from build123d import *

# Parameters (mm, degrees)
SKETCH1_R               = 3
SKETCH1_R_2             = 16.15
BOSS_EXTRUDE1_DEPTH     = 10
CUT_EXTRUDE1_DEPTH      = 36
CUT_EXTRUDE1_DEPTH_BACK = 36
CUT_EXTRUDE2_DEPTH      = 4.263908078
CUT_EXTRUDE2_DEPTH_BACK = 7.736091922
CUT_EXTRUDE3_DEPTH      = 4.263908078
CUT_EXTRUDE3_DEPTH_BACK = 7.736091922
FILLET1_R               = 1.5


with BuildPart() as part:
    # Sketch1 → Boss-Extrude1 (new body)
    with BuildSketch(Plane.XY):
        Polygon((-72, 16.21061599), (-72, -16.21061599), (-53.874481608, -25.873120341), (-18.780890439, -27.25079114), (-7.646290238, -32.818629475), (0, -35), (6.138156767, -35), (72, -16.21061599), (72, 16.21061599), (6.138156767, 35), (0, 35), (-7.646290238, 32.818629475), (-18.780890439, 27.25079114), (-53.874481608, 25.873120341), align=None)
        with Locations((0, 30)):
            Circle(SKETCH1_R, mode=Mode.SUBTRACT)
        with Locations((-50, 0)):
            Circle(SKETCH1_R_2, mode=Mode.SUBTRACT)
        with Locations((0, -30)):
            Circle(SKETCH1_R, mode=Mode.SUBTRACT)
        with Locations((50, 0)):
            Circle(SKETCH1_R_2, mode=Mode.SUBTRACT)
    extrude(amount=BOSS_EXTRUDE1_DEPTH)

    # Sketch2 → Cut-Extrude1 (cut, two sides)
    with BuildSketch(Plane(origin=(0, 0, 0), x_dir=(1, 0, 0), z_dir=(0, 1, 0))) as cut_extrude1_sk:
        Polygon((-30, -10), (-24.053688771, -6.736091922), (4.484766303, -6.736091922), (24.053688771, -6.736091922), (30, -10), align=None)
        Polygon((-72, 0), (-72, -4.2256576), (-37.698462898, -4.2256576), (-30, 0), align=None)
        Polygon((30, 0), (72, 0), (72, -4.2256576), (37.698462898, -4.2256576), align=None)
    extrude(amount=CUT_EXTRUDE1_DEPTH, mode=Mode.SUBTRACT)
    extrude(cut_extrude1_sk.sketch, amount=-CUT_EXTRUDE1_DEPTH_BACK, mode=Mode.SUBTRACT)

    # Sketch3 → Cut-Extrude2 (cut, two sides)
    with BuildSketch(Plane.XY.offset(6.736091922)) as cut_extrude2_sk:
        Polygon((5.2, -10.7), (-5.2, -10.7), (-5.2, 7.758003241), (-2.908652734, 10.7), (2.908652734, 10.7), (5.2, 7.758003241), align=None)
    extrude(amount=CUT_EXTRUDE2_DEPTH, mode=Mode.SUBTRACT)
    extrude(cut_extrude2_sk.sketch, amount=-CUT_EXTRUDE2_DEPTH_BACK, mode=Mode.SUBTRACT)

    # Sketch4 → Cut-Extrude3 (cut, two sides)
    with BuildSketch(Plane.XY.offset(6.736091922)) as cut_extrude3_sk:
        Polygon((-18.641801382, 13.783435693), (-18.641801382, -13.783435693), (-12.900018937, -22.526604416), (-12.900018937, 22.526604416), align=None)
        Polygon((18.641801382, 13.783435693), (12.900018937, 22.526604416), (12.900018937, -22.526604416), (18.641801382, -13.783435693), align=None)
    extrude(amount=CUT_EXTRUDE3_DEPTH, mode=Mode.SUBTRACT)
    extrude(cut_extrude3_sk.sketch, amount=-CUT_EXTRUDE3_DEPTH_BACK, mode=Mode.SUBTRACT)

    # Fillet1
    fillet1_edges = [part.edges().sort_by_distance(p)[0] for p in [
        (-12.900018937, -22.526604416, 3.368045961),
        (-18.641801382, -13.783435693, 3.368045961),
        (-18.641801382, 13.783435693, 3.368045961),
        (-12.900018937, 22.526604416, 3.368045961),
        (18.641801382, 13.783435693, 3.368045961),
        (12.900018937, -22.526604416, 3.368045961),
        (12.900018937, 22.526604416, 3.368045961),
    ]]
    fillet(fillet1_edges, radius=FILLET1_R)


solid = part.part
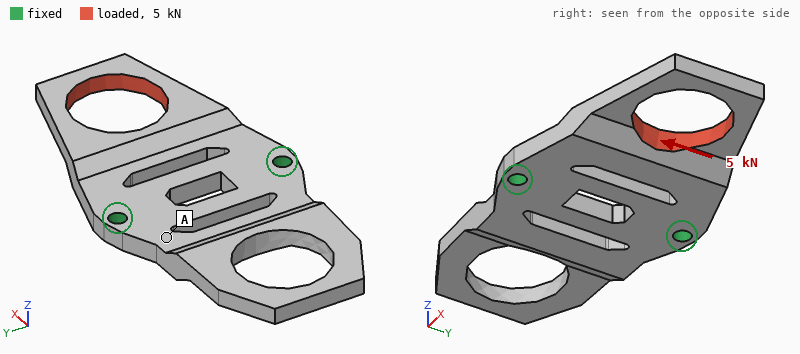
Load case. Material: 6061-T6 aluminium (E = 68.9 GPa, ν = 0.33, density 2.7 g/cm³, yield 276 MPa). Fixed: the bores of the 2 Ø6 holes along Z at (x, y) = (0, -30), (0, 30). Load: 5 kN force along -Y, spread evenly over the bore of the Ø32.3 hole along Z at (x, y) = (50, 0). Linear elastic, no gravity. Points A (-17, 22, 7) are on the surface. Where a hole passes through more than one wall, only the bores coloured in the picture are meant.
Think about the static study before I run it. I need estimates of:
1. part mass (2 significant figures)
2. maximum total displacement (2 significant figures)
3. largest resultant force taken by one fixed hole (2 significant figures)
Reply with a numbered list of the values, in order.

1. 98 g
2. 0.22 mm
3. 4.5 kN
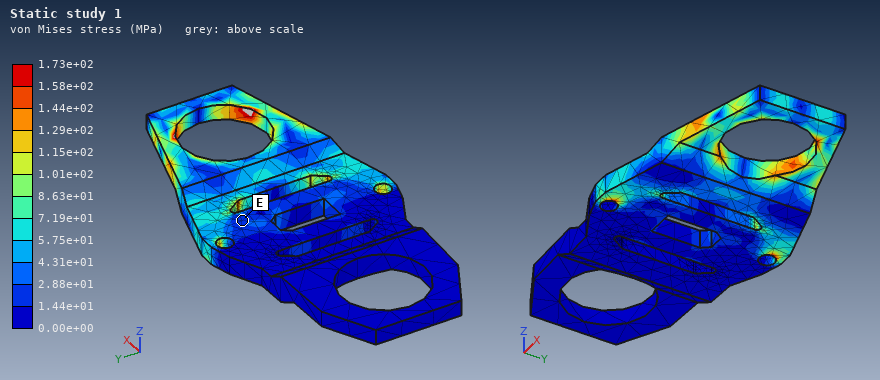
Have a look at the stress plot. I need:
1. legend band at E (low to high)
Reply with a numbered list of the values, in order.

1. 1.44e+01 to 2.88e+01 MPa
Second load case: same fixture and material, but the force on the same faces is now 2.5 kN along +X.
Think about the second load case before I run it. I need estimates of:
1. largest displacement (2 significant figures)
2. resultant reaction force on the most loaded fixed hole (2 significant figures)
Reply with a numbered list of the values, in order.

1. 0.26 mm
2. 1.3 kN
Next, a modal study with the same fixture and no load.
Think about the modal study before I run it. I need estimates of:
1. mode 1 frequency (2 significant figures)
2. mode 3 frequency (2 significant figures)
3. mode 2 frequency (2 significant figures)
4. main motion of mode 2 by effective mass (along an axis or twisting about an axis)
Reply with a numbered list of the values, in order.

1. 1100 Hz
2. 3600 Hz
3. 1300 Hz
4. along Z
